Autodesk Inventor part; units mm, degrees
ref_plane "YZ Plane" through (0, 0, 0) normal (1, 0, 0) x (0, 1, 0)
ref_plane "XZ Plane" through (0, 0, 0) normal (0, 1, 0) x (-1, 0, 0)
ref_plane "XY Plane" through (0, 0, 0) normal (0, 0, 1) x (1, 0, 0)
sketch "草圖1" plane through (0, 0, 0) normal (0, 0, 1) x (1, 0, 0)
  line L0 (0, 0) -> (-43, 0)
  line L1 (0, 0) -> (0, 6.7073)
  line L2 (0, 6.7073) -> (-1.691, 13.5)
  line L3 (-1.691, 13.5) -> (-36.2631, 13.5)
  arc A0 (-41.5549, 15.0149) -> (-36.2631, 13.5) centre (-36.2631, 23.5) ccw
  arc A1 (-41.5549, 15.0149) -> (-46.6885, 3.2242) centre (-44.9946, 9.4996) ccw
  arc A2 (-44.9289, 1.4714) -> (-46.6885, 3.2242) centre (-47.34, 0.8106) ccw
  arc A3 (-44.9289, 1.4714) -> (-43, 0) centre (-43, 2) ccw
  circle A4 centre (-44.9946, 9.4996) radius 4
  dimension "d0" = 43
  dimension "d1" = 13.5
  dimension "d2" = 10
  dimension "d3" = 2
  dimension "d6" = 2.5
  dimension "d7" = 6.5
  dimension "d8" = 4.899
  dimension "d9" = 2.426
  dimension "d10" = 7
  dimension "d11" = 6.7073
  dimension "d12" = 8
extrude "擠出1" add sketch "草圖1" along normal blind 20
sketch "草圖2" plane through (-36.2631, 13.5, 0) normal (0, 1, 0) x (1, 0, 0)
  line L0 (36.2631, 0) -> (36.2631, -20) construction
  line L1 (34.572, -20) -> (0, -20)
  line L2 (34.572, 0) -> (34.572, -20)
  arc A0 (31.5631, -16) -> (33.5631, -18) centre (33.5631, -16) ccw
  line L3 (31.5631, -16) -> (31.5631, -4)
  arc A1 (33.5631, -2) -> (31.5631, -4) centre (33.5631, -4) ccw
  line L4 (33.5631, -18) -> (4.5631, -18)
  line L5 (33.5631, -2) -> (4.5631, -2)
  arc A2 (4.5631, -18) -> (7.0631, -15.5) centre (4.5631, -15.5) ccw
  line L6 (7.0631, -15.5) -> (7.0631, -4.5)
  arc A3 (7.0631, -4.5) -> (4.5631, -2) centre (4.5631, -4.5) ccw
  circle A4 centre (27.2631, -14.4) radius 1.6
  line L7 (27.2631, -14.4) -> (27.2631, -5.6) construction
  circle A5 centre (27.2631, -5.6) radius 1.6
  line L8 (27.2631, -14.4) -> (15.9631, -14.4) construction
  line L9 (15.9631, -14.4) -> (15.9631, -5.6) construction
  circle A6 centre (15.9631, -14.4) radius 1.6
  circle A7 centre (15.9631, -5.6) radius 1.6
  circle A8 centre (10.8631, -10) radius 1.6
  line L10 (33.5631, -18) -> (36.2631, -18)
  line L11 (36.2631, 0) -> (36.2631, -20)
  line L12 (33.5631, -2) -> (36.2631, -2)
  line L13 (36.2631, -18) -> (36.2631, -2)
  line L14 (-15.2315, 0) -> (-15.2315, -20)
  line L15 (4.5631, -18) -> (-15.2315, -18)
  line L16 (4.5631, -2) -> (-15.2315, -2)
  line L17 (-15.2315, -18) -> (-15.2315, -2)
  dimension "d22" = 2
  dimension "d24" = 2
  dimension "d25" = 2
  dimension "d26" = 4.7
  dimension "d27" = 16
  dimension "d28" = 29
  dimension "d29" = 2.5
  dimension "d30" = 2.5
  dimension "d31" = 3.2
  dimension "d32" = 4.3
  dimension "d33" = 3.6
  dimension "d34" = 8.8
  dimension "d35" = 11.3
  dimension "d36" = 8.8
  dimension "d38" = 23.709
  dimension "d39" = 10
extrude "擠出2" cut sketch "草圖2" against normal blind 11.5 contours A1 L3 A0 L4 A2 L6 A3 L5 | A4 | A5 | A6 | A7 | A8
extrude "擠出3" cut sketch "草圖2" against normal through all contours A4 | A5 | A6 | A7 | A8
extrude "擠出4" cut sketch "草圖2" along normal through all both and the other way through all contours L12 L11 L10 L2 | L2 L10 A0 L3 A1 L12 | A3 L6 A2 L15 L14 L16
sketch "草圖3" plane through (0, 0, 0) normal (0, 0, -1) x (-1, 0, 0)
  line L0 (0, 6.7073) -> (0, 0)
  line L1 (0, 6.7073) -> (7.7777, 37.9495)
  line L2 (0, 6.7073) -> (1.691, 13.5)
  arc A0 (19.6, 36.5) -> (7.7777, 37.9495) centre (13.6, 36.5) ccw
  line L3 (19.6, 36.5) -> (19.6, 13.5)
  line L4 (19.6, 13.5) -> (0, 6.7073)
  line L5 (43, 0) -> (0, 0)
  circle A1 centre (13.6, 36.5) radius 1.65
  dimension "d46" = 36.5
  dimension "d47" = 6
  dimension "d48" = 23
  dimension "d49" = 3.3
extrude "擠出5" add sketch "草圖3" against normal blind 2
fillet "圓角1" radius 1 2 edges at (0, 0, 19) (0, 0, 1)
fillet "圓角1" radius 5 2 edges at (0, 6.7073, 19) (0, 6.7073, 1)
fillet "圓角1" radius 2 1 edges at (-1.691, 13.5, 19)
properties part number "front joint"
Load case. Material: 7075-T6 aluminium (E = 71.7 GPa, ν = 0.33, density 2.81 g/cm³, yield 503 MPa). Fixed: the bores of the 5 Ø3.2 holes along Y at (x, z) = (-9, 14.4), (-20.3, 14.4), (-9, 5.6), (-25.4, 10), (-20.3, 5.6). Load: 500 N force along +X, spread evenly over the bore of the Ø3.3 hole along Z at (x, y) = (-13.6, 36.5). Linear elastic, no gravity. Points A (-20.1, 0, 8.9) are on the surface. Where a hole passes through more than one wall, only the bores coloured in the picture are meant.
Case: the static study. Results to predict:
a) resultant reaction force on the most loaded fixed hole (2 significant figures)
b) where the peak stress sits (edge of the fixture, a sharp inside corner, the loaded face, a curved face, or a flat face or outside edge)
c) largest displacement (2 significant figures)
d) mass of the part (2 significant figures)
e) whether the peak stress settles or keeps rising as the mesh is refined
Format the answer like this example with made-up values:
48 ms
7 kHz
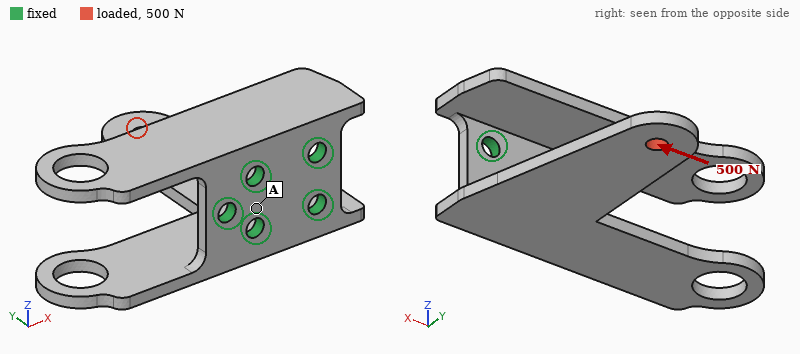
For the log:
1.3 kN
edge of the fixture
0.41 mm
11 g
keeps rising
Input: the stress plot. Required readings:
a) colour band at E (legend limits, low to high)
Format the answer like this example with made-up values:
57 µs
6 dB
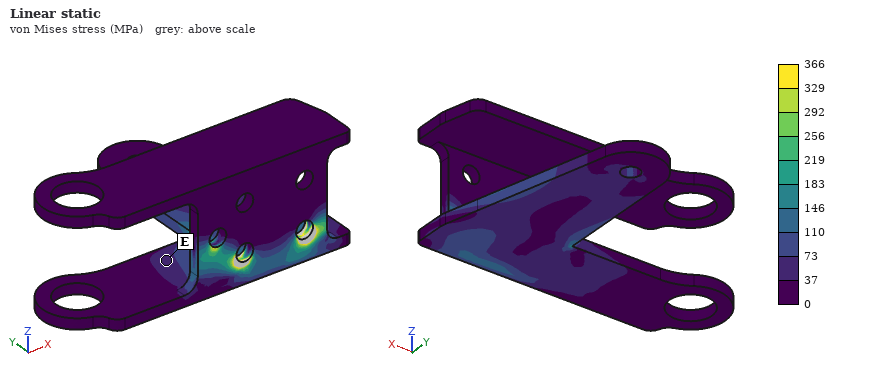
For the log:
37 to 73 MPa
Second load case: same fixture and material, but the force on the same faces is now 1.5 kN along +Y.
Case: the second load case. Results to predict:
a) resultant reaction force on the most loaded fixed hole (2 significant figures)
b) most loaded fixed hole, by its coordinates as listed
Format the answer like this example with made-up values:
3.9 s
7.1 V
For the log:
900 N
(-9, 5.6)
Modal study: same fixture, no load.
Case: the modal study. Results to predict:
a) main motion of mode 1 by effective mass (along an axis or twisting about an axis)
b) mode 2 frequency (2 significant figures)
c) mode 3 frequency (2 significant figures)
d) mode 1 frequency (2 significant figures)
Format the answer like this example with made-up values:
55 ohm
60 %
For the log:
along Z
2800 Hz
2800 Hz
1200 Hz
